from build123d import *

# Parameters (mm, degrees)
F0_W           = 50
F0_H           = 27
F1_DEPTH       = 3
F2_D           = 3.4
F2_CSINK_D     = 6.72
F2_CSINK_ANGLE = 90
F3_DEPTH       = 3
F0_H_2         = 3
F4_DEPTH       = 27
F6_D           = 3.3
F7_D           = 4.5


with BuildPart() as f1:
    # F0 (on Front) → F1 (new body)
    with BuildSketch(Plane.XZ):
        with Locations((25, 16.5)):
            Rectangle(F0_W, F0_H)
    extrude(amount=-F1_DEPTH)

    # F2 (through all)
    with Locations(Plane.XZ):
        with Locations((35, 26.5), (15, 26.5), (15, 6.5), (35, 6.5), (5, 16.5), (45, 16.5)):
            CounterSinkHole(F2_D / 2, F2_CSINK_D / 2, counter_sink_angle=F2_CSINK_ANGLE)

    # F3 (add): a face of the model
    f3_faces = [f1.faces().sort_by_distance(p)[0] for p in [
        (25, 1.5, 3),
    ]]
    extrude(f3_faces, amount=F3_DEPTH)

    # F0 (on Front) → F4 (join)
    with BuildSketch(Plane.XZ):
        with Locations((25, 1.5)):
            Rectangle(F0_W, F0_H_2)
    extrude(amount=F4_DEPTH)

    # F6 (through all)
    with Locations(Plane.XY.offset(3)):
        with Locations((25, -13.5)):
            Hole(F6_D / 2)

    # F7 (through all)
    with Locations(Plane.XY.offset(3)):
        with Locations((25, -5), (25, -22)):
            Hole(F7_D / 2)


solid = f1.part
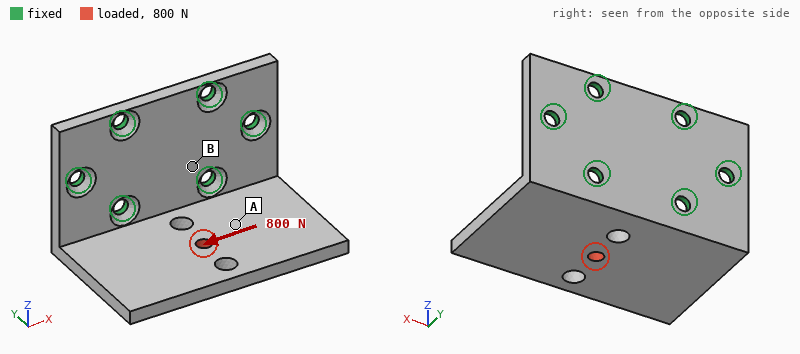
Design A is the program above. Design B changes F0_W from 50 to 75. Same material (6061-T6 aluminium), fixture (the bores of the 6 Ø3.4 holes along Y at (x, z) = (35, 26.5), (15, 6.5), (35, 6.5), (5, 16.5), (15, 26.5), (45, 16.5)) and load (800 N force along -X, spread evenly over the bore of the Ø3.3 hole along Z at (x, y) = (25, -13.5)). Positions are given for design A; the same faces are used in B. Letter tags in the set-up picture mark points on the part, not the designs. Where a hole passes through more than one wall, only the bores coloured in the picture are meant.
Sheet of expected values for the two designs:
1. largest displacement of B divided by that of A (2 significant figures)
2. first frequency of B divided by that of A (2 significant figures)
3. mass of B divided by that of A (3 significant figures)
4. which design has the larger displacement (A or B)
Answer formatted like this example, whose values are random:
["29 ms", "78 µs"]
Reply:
["1.1", "0.97", "1.52", "B"]
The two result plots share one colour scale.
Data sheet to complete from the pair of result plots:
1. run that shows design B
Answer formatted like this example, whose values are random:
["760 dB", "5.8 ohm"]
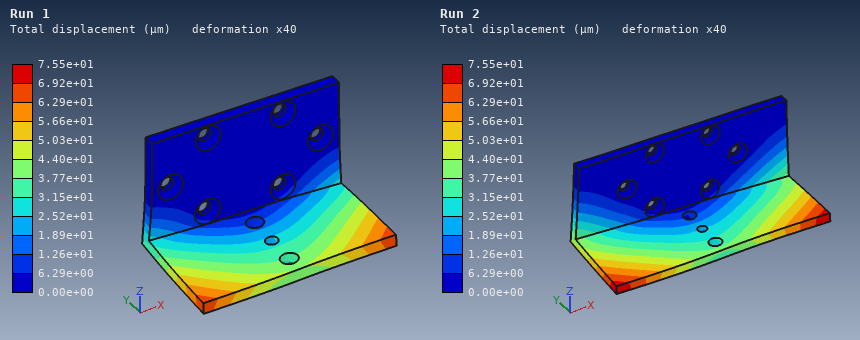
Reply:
["Run 2"]
